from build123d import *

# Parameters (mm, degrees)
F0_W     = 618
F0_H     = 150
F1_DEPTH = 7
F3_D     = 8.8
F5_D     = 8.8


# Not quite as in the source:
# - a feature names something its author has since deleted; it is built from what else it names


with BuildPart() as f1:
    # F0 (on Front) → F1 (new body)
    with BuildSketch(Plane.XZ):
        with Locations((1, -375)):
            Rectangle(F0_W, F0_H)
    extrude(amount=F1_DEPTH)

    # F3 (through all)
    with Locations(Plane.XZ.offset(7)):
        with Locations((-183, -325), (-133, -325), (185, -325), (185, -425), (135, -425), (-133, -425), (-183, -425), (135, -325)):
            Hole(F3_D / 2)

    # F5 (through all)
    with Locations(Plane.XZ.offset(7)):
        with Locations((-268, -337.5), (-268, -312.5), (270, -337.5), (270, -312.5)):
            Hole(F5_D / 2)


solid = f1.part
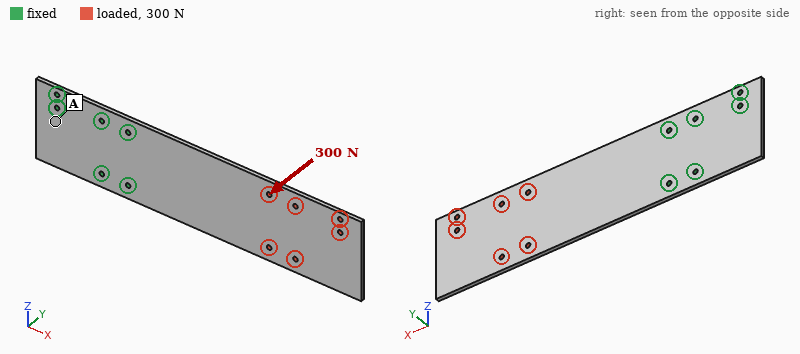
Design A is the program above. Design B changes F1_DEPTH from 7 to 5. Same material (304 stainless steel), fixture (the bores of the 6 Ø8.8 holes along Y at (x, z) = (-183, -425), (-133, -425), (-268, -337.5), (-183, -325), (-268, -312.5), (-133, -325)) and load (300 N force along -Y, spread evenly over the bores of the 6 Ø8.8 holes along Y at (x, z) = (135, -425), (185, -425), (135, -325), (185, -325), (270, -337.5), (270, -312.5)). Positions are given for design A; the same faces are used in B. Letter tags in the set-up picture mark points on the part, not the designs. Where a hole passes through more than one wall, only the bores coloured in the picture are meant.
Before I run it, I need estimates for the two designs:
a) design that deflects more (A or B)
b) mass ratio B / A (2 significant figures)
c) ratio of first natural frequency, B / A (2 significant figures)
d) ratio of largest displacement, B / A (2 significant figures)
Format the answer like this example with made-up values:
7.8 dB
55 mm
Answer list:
B
0.71
0.72
2.7
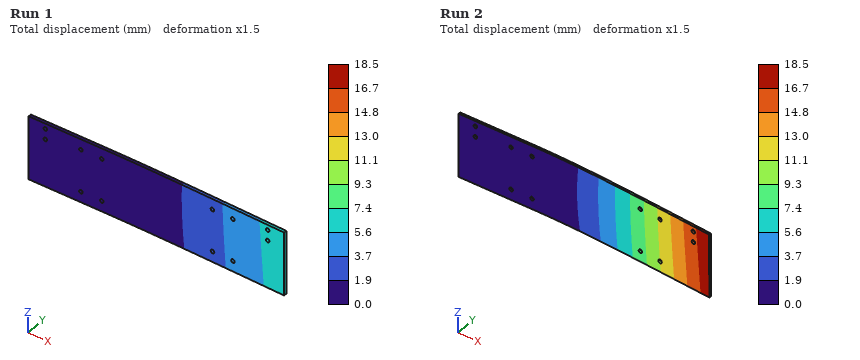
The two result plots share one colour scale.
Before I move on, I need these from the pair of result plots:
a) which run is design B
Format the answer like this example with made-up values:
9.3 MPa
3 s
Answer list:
Run 2
